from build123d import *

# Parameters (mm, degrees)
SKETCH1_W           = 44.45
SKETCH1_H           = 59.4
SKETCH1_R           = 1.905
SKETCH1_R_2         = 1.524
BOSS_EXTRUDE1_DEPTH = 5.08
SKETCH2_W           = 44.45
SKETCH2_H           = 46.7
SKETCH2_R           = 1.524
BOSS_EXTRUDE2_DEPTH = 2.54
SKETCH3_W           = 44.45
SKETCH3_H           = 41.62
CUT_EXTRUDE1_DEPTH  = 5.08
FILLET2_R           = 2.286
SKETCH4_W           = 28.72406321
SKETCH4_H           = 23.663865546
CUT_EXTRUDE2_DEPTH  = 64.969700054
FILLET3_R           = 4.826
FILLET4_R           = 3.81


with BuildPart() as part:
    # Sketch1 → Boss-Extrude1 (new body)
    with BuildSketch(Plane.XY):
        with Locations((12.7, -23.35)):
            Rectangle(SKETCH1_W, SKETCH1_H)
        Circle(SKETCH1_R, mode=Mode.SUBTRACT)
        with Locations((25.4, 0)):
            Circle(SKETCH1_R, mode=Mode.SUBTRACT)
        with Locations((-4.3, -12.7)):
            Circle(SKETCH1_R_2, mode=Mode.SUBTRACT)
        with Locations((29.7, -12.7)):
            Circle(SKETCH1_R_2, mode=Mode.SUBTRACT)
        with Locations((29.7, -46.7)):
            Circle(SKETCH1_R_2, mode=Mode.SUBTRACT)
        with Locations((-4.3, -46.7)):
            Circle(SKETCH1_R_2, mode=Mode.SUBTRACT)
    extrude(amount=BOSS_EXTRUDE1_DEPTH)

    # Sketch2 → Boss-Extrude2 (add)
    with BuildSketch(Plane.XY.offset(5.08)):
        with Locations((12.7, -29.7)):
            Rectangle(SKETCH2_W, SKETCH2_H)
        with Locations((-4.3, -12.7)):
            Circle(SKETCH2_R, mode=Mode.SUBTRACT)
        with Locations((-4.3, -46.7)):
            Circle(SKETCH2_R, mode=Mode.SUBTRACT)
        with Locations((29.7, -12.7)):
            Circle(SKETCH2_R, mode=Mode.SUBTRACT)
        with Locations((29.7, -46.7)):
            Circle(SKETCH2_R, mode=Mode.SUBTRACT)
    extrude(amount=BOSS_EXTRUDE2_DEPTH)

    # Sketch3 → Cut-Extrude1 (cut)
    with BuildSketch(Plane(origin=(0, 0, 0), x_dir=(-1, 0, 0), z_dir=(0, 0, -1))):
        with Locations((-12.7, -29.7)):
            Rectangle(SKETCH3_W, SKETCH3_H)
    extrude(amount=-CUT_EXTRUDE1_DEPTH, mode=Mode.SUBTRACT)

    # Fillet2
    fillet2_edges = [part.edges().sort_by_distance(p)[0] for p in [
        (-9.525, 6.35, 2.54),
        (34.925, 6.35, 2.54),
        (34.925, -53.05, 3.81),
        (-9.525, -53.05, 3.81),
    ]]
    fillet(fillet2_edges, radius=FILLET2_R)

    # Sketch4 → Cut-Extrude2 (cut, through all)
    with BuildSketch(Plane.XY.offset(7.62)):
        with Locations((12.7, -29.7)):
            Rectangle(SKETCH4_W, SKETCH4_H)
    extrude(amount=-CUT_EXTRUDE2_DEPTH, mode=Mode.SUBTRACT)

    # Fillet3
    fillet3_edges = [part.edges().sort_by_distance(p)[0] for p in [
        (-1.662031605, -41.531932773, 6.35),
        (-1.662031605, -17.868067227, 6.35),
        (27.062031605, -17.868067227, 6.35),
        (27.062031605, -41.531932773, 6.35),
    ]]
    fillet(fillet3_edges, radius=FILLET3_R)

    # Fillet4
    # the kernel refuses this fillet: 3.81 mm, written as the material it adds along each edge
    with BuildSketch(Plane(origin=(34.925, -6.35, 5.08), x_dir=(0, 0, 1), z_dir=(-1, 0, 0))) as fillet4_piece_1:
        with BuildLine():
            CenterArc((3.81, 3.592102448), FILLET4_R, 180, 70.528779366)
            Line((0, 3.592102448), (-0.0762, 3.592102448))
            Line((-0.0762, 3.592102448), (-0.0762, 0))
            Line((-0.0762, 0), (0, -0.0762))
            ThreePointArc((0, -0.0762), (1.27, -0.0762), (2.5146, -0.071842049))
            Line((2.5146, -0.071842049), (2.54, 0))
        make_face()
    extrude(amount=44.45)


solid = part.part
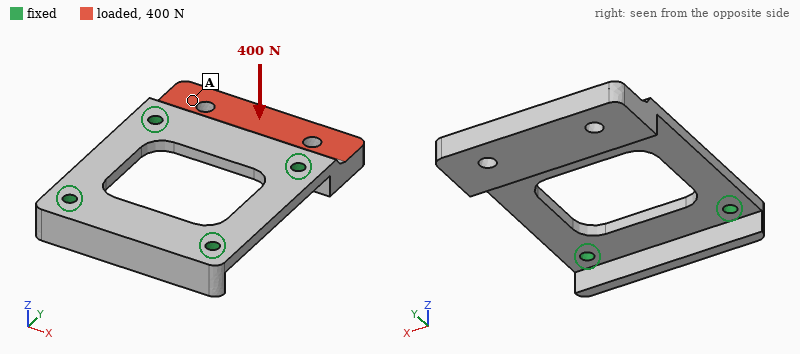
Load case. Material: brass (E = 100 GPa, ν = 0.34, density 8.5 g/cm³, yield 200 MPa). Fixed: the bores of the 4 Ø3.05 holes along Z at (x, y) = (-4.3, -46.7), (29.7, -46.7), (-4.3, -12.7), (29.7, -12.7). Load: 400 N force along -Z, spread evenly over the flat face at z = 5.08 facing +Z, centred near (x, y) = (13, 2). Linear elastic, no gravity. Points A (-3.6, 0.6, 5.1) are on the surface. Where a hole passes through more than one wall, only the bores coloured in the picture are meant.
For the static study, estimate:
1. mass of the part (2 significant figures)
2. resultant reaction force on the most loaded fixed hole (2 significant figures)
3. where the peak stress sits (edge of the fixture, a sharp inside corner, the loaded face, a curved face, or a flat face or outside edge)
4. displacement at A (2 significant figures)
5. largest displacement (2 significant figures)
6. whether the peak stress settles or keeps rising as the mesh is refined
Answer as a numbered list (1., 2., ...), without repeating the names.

1. 64 g
2. 230 N
3. edge of the fixture
4. 0.063 mm
5. 0.11 mm
6. keeps rising
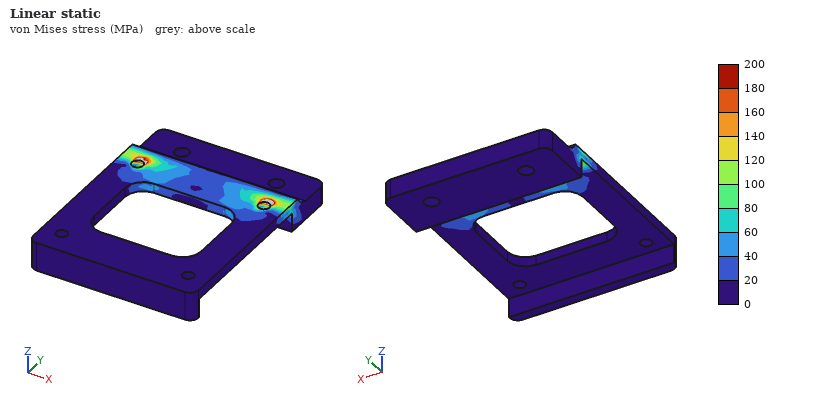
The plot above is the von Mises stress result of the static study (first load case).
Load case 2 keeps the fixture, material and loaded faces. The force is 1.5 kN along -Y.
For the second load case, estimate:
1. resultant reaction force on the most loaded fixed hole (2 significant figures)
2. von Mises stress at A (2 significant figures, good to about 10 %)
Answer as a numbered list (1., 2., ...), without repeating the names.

1. 750 N
2. 24 MPa
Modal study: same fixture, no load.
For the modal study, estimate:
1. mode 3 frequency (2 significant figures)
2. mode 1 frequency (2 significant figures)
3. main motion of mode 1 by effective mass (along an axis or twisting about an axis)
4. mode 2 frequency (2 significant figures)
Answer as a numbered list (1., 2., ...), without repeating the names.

1. 8700 Hz
2. 2500 Hz
3. along Z
4. 6700 Hz
